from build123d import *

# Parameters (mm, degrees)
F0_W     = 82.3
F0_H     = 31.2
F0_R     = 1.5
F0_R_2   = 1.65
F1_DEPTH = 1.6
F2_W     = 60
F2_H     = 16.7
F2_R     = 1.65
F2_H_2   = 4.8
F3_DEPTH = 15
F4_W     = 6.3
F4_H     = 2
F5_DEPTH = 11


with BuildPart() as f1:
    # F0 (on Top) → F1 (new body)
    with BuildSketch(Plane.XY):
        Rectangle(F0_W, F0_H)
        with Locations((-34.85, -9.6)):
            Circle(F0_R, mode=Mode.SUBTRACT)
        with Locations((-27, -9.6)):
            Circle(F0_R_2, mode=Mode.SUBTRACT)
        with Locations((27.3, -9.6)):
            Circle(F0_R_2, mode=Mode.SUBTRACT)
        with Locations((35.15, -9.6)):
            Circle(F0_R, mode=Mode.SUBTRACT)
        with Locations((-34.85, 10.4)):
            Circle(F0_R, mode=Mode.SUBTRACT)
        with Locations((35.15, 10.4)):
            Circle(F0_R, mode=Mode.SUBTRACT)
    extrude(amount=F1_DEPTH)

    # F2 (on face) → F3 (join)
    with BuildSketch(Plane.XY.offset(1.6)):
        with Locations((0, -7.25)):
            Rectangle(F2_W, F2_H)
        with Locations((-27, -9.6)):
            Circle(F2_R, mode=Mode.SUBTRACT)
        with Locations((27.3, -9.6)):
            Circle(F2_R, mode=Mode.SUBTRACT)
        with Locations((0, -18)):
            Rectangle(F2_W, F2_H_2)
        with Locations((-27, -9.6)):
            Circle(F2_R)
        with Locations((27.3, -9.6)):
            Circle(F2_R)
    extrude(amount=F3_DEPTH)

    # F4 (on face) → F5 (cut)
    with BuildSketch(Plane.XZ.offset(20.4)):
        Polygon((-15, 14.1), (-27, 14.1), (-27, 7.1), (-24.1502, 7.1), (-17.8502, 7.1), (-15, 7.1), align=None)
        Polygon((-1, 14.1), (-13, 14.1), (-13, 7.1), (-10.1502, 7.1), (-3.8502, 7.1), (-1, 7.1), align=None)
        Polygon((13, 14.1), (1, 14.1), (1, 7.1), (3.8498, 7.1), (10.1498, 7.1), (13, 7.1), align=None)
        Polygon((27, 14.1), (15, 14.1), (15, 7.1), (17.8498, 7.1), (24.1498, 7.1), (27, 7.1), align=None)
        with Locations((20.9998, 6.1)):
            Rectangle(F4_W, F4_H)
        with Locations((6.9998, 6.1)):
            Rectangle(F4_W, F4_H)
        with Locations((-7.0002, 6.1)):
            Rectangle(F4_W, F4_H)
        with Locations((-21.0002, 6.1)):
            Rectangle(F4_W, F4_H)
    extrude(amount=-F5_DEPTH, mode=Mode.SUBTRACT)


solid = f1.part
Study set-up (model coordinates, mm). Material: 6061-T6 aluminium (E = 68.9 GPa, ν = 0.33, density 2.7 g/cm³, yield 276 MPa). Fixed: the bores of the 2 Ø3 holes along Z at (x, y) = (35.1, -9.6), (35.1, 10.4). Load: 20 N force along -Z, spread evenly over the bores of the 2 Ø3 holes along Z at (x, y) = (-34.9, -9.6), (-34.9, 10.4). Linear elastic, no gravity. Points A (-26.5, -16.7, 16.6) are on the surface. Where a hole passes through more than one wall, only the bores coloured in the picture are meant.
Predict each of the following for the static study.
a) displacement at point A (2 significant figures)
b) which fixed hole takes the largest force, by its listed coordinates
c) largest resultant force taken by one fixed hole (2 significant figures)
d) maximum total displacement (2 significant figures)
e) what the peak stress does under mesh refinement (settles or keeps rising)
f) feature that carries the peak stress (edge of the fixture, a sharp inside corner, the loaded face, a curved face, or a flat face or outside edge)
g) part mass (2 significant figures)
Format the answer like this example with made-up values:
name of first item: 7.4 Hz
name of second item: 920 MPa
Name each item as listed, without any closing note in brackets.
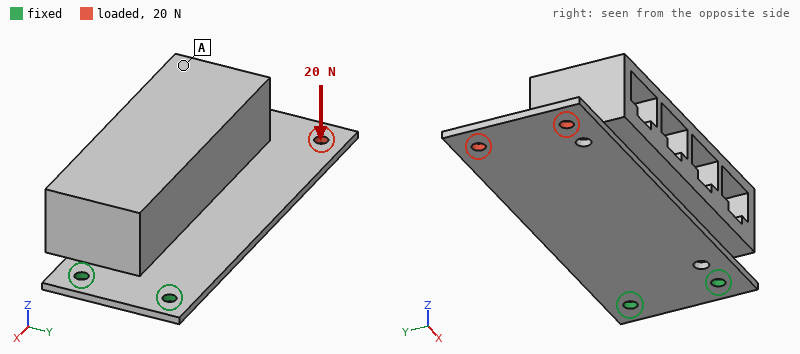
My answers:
displacement at point A: 0.72 mm
which fixed hole takes the largest force, by its listed coordinates: (35.1, 10.4)
largest resultant force taken by one fixed hole: 15 N
maximum total displacement: 0.89 mm
what the peak stress does under mesh refinement: keeps rising
feature that carries the peak stress: edge of the fixture
part mass: 52 g
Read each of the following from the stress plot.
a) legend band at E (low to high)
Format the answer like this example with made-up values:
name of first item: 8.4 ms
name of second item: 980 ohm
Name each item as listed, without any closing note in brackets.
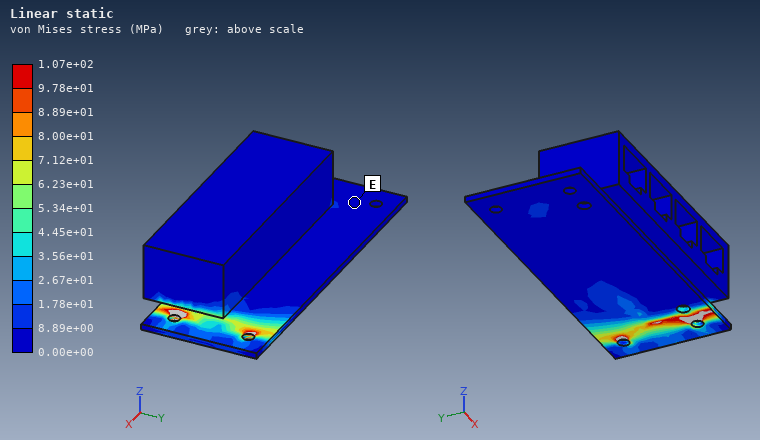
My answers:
legend band at E: 0.00e+00 to 8.89e+00 MPa
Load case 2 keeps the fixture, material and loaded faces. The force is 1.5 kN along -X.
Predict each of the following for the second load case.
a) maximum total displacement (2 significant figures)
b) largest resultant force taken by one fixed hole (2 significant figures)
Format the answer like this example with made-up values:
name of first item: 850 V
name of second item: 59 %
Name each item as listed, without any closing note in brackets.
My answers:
maximum total displacement: 86 µm
largest resultant force taken by one fixed hole: 760 N
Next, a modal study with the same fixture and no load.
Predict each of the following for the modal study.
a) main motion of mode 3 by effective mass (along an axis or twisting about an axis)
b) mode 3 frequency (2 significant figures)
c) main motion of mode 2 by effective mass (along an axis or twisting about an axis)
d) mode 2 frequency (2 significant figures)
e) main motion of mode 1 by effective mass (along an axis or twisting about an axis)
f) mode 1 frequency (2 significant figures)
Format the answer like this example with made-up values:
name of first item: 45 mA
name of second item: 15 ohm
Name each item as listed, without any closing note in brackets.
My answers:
main motion of mode 3 by effective mass: along Y
mode 3 frequency: 2600 Hz
main motion of mode 2 by effective mass: along Y
mode 2 frequency: 1500 Hz
main motion of mode 1 by effective mass: along Z
mode 1 frequency: 190 Hz
